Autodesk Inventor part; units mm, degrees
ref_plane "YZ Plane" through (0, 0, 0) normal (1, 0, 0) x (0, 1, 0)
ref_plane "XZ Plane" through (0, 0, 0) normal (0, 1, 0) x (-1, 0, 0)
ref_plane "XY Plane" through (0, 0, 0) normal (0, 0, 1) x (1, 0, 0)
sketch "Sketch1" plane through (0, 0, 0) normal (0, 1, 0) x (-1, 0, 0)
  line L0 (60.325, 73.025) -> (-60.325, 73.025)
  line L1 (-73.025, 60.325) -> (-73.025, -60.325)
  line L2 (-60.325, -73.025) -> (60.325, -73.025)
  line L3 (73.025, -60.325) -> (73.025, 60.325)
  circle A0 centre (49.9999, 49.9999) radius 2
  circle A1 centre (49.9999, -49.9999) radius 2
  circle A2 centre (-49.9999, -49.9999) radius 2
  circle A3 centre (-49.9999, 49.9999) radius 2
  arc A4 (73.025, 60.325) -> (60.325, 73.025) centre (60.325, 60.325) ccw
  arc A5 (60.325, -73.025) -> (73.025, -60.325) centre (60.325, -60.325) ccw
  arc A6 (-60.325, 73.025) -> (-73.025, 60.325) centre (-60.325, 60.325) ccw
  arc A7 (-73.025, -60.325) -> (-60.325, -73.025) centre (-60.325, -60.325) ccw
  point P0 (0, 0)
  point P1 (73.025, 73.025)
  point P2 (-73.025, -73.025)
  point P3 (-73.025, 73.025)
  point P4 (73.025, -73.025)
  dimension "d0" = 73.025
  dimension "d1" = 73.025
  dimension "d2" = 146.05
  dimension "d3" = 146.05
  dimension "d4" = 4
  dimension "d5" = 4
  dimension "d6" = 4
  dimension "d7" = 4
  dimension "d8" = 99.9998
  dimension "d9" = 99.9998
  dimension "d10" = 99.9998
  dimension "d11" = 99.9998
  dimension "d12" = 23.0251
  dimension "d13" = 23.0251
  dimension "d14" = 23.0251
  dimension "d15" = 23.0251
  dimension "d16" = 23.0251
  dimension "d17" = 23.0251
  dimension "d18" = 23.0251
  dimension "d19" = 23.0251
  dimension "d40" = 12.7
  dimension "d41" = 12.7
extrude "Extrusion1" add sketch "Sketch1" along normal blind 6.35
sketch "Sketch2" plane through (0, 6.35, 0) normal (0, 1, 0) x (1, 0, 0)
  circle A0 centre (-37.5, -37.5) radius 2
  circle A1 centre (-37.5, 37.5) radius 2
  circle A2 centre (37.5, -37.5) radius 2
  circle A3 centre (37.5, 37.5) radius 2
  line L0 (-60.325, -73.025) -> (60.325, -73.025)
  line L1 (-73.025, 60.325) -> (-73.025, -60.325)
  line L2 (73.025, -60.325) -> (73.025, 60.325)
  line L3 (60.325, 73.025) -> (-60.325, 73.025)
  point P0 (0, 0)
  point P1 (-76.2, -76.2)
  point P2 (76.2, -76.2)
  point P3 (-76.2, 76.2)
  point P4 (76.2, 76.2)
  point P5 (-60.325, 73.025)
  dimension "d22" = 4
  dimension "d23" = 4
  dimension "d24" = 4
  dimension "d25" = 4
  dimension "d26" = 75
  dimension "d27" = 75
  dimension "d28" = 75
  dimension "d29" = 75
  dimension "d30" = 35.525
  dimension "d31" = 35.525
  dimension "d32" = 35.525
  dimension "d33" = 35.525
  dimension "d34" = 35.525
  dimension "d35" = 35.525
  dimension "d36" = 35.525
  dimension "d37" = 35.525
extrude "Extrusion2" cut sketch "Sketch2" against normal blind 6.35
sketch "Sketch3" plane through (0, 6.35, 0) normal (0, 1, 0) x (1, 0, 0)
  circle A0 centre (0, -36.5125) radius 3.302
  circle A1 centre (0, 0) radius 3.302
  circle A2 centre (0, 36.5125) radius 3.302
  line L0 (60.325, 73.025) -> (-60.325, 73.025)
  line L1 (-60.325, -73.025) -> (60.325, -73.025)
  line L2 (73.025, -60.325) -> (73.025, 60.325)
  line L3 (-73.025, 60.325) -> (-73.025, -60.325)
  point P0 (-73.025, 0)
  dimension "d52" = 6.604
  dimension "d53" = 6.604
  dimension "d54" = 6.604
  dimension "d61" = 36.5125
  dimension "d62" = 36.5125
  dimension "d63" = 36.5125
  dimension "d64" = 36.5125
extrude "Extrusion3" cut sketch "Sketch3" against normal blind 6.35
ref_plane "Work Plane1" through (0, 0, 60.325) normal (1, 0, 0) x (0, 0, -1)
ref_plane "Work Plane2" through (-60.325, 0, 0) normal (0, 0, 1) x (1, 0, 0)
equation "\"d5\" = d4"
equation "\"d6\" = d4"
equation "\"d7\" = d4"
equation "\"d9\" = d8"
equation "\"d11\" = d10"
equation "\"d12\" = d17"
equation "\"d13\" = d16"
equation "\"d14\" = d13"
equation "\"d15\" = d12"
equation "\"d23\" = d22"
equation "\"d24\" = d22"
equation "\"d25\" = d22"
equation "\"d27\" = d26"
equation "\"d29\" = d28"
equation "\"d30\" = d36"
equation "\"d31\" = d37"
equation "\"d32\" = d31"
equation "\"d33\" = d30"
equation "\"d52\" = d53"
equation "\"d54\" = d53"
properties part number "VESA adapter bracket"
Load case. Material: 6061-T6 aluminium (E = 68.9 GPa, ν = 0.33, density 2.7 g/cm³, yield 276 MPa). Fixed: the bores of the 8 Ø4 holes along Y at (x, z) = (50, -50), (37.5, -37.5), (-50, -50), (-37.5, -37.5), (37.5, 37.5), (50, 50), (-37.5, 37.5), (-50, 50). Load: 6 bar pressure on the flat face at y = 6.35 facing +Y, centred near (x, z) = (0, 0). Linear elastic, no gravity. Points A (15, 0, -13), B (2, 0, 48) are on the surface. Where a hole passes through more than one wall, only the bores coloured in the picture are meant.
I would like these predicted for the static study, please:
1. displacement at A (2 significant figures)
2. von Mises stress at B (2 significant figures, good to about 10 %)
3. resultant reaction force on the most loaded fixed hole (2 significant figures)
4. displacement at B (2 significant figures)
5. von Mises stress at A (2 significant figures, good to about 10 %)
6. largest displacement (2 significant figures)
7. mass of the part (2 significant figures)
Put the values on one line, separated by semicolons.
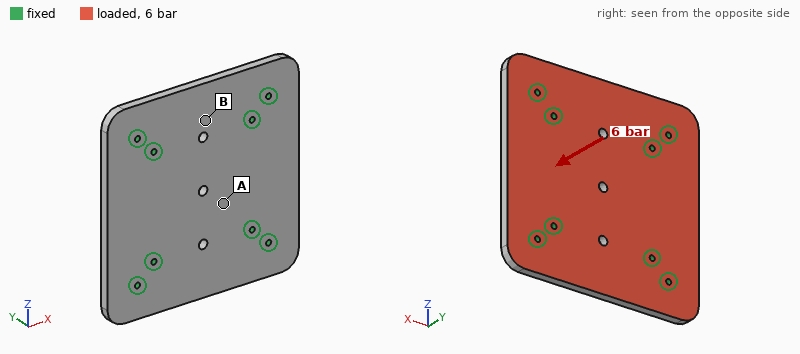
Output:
64 µm; 29 MPa; 2.2 kN; 60 µm; 14 MPa; 91 µm; 360 g
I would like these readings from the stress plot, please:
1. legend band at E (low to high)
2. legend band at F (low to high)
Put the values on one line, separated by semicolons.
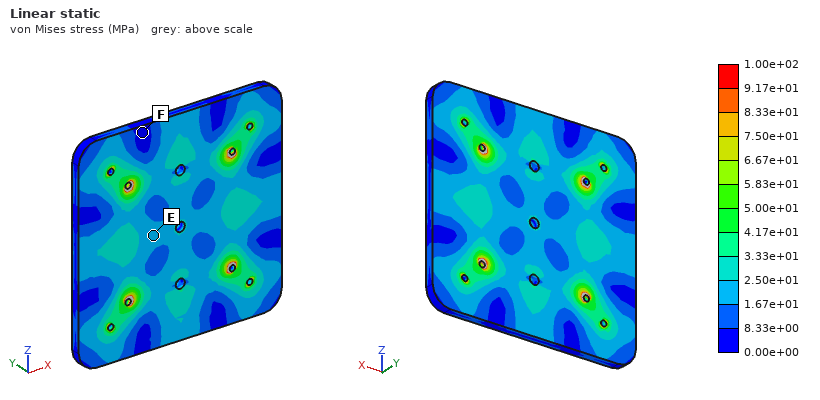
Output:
1.67e+01 to 2.50e+01 MPa; 0.00e+00 to 8.33e+00 MPa
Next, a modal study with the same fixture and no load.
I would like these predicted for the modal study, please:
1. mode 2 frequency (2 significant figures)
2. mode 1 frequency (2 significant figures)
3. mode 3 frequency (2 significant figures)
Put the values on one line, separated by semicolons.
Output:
3700 Hz; 3300 Hz; 3700 Hz
